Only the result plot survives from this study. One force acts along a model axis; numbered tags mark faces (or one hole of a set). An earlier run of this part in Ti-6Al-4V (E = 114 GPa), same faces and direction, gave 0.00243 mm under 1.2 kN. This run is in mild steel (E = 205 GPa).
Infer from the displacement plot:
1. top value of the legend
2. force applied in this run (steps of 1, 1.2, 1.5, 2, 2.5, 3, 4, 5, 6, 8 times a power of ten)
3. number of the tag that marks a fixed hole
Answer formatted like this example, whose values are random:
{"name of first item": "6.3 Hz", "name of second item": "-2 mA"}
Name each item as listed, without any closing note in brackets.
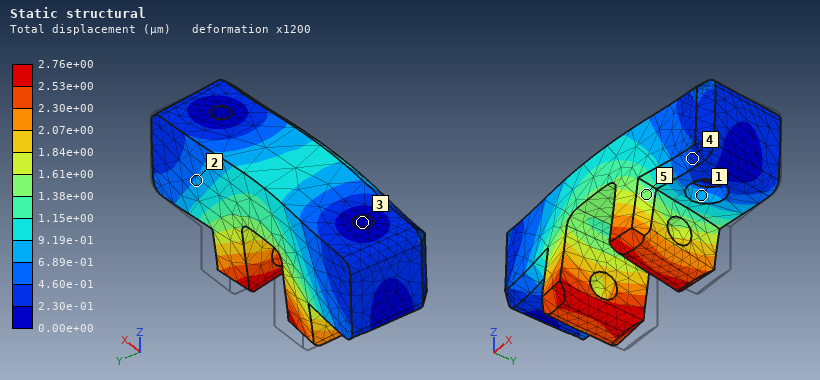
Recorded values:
{"top value of the legend": "2.76e+00 µm", "force applied in this run": "2.5 kN", "number of the tag that marks a fixed hole": "3"}
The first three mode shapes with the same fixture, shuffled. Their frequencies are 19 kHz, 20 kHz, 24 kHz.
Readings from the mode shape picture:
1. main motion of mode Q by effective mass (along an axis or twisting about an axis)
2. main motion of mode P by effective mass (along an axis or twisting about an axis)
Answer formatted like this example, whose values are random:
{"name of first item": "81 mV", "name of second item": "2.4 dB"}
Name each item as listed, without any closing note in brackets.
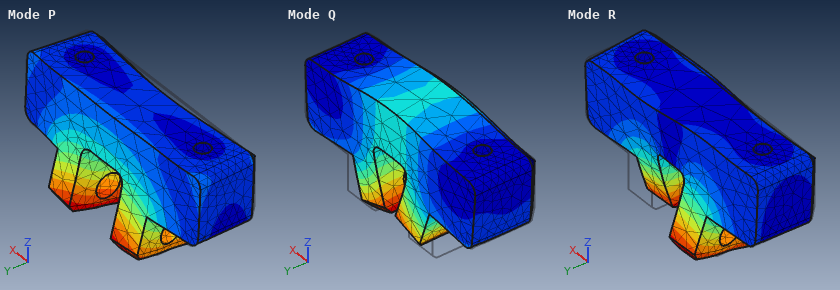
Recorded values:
{"main motion of mode Q by effective mass": "along Z", "main motion of mode P by effective mass": "along Y"}
